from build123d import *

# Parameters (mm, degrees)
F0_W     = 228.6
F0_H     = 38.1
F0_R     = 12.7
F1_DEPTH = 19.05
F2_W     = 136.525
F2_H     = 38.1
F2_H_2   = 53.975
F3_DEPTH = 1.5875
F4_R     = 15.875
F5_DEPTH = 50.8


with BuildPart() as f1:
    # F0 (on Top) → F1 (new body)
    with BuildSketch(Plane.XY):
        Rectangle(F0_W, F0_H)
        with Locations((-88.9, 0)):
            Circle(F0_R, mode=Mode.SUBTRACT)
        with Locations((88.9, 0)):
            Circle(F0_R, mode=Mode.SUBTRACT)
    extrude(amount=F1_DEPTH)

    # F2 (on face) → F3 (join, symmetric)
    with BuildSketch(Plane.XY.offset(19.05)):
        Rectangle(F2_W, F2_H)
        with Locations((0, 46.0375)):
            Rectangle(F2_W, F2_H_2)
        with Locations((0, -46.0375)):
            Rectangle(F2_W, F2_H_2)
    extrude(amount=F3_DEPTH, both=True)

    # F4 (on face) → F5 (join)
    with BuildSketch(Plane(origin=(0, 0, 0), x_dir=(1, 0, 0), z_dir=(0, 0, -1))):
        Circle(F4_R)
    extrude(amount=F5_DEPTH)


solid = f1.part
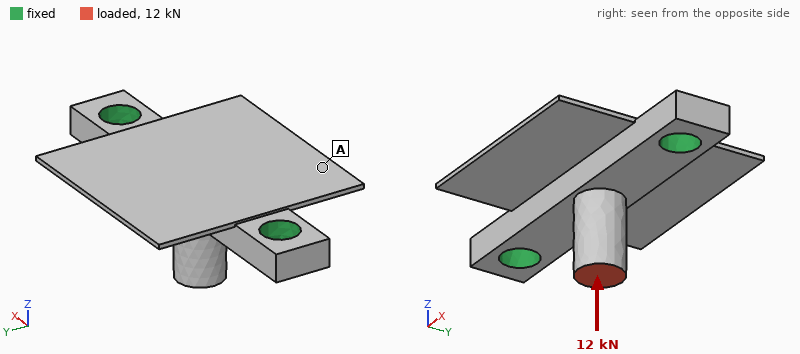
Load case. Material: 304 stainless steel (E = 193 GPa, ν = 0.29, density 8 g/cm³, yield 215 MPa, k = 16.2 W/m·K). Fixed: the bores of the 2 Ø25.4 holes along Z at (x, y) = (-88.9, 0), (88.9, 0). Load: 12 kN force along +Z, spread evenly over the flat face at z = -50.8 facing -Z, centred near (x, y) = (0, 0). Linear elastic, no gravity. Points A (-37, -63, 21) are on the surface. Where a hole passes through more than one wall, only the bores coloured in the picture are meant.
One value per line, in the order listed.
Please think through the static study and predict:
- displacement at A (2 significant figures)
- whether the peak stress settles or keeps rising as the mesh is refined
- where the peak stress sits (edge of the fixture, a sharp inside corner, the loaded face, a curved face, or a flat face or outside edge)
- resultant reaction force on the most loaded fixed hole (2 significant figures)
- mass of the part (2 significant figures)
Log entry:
35 µm
keeps rising
edge of the fixture
6.2 kN
1.9 kg
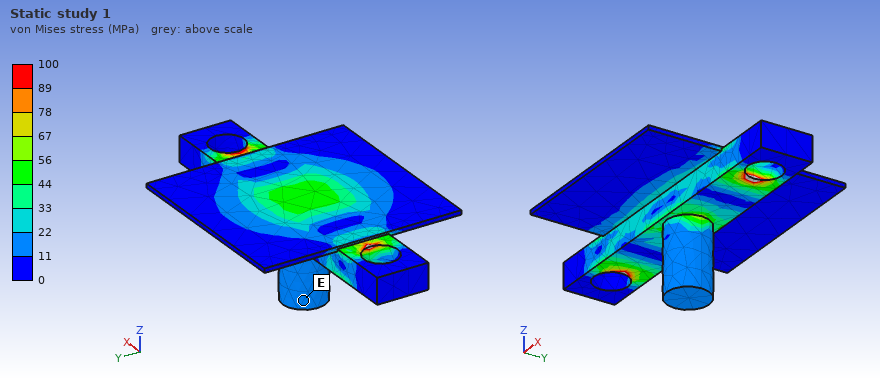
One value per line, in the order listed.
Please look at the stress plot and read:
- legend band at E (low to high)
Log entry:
11 to 22 MPa
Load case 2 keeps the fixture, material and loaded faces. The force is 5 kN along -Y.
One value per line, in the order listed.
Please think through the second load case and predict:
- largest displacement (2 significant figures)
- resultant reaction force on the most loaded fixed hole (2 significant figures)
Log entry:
0.16 mm
2.5 kN
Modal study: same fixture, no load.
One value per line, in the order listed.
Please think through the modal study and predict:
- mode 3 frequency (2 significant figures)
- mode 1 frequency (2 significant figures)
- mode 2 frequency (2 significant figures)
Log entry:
1200 Hz
840 Hz
870 Hz
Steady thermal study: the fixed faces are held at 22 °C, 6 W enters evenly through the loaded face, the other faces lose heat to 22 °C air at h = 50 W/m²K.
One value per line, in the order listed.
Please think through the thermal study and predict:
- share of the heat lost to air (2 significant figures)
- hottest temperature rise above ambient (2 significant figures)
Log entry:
87 %
21 K
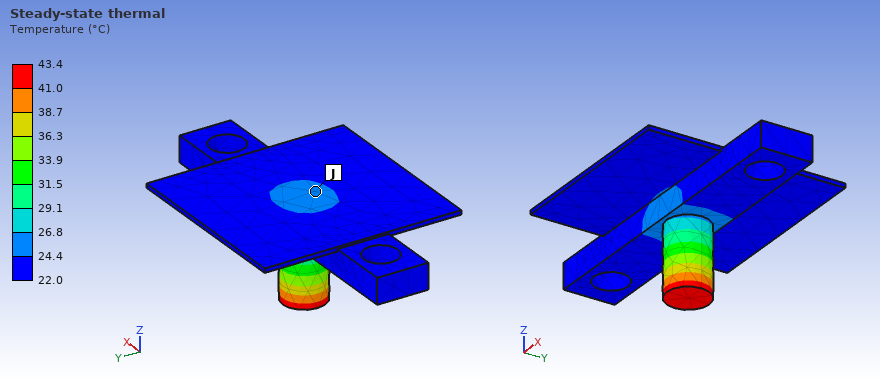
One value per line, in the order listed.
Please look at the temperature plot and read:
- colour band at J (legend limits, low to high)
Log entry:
24.4 to 26.8 °C
